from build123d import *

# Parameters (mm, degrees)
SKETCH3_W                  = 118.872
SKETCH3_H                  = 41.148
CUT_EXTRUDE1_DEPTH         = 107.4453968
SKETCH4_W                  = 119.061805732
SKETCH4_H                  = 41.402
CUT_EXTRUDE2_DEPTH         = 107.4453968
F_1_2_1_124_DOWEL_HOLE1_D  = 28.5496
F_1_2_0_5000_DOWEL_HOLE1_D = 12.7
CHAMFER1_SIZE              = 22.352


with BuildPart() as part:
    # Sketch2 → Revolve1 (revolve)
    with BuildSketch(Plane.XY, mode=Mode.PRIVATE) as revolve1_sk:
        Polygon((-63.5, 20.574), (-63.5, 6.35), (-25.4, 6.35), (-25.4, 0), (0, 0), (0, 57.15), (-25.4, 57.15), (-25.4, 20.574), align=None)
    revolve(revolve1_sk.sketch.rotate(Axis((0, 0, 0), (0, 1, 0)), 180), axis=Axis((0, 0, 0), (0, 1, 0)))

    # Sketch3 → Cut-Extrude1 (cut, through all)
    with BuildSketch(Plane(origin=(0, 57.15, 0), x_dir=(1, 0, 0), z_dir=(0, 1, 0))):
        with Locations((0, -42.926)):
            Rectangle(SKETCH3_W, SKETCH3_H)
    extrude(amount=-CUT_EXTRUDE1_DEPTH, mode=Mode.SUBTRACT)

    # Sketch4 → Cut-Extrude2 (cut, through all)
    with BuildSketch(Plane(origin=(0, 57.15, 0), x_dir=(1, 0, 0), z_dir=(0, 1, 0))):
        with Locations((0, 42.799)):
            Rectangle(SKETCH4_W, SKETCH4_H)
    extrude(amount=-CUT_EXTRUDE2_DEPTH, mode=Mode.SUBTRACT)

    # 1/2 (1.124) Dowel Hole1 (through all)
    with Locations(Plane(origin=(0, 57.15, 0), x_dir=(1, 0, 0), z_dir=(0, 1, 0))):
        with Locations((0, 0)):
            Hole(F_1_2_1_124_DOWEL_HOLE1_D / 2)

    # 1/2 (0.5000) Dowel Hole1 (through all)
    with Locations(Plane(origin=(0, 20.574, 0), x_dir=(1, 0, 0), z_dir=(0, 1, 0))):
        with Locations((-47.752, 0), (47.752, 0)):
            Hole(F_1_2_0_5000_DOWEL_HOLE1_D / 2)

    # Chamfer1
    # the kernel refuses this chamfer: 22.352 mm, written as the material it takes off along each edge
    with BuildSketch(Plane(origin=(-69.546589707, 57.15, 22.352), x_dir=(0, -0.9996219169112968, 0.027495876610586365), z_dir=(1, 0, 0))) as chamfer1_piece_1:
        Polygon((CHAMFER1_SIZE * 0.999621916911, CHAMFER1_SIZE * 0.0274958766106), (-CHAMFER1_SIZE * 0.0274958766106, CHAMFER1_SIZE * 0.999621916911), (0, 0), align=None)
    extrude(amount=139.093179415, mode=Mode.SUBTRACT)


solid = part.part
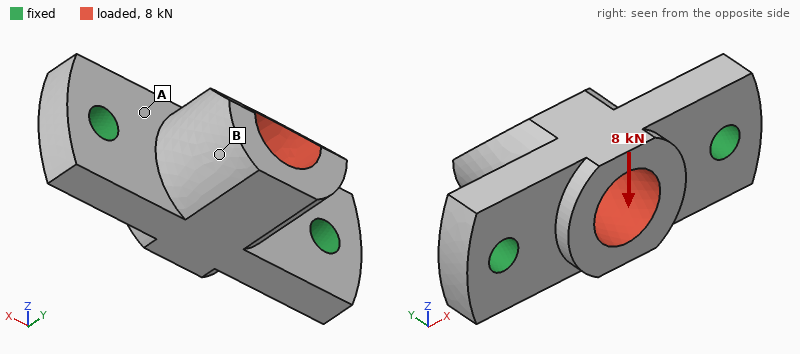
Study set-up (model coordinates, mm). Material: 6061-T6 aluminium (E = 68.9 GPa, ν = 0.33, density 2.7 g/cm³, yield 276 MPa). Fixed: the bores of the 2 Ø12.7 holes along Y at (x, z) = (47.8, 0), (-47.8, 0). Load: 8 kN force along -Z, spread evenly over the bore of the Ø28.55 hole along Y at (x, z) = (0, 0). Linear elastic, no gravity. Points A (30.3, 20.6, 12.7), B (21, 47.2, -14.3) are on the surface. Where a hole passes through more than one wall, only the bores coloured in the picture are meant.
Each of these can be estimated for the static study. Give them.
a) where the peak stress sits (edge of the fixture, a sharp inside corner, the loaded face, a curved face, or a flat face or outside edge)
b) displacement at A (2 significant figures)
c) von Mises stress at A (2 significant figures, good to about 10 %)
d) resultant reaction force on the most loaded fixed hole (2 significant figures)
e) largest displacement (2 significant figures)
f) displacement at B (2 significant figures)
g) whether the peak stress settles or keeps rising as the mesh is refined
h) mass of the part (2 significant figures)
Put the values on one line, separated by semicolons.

edge of the fixture; 17 µm; 32 MPa; 4.0 kN; 86 µm; 65 µm; keeps rising; 310 g
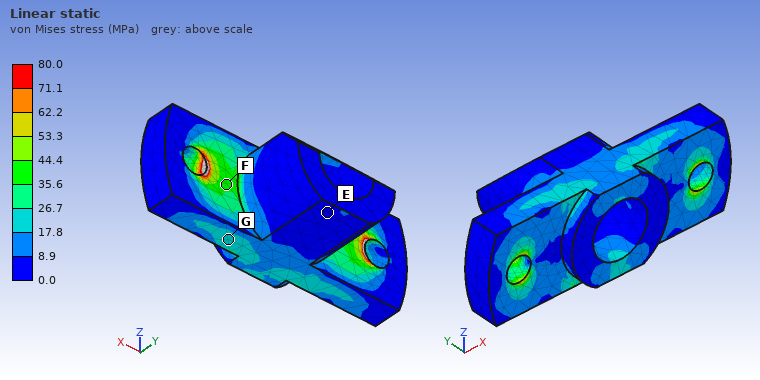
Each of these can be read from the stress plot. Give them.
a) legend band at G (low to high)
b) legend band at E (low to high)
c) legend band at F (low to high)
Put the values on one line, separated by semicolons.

17.8 to 26.7 MPa; 0.0 to 8.9 MPa; 35.6 to 44.4 MPa
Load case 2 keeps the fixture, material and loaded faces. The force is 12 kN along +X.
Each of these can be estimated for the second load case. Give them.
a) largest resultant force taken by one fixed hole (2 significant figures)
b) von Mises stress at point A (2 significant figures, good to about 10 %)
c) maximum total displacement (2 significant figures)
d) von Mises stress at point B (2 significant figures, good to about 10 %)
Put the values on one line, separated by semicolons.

6.4 kN; 16 MPa; 31 µm; 4.3 MPa
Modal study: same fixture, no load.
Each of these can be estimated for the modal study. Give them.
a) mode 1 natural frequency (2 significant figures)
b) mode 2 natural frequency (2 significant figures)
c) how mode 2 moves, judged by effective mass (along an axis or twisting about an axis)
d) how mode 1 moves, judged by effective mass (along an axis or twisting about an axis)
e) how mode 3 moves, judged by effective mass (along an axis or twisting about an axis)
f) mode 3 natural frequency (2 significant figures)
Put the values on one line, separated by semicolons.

4100 Hz; 6800 Hz; along Y; along Z; along X; 8700 Hz
